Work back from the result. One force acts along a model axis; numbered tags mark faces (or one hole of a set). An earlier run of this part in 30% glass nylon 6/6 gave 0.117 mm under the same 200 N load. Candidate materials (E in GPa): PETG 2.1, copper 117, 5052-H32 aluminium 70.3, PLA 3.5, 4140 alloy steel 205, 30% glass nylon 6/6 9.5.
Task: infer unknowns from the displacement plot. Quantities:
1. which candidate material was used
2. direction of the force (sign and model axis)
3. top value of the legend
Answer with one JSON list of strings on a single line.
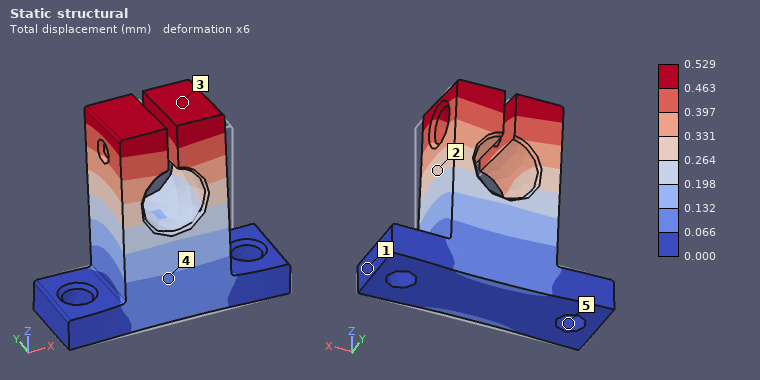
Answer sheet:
["PETG", "+Y", "0.529 mm"]
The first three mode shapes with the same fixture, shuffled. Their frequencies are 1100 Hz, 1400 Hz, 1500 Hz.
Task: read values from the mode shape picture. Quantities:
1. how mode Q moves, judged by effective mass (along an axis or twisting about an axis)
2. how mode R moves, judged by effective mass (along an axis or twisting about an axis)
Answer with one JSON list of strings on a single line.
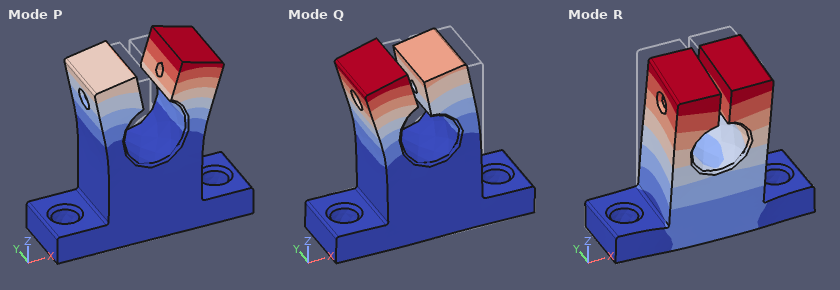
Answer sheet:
["along X", "along Y"]
